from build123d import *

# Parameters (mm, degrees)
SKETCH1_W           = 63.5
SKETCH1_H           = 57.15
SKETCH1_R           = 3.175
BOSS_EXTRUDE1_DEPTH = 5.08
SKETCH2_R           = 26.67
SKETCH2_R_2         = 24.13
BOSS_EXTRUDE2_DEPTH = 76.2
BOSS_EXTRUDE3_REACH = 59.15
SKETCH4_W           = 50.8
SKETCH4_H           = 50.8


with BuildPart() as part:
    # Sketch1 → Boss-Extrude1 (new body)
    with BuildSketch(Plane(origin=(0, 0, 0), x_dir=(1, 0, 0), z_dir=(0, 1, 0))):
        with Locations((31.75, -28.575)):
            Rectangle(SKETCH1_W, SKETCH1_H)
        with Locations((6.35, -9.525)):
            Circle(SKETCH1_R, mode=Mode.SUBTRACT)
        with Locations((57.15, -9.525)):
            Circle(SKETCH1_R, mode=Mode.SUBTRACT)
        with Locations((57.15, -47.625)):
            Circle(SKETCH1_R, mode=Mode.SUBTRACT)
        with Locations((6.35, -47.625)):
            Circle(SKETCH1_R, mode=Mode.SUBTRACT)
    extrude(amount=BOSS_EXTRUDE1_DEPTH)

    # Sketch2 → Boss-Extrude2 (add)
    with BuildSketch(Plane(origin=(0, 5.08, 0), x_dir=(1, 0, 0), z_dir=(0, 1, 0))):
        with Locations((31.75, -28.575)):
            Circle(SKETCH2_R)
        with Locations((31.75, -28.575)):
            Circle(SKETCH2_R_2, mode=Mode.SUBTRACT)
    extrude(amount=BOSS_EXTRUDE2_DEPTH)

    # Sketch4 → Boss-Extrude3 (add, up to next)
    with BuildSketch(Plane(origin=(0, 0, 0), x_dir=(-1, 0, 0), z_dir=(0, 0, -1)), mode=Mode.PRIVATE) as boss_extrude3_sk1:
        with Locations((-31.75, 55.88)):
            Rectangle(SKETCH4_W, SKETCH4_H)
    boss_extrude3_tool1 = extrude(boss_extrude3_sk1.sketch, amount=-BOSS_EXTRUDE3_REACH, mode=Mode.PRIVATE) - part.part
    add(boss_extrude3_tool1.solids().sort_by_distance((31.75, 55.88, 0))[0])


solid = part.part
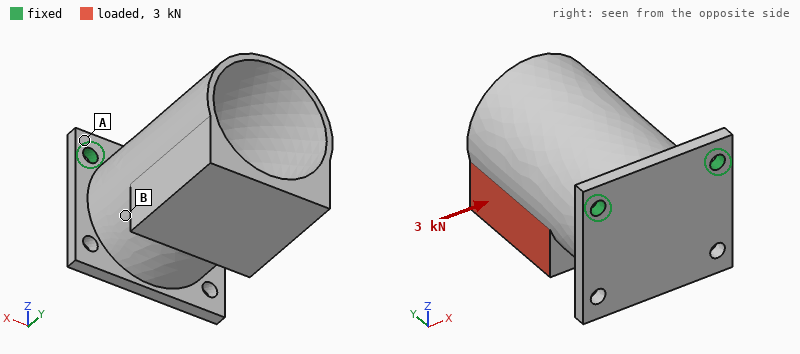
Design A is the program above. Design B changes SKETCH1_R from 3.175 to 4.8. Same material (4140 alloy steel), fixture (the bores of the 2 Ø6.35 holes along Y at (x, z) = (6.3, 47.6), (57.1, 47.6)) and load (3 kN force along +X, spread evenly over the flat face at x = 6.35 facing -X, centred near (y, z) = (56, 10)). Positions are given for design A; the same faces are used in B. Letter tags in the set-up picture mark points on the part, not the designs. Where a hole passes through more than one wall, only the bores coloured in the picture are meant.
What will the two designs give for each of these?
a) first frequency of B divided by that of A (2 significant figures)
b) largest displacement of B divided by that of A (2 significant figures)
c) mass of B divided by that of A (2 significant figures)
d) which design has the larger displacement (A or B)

1.2
0.89
0.99
A
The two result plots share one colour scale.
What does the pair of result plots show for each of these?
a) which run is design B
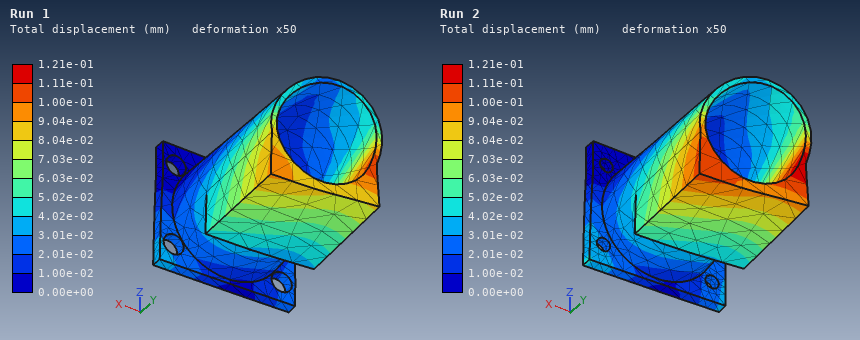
Run 1
